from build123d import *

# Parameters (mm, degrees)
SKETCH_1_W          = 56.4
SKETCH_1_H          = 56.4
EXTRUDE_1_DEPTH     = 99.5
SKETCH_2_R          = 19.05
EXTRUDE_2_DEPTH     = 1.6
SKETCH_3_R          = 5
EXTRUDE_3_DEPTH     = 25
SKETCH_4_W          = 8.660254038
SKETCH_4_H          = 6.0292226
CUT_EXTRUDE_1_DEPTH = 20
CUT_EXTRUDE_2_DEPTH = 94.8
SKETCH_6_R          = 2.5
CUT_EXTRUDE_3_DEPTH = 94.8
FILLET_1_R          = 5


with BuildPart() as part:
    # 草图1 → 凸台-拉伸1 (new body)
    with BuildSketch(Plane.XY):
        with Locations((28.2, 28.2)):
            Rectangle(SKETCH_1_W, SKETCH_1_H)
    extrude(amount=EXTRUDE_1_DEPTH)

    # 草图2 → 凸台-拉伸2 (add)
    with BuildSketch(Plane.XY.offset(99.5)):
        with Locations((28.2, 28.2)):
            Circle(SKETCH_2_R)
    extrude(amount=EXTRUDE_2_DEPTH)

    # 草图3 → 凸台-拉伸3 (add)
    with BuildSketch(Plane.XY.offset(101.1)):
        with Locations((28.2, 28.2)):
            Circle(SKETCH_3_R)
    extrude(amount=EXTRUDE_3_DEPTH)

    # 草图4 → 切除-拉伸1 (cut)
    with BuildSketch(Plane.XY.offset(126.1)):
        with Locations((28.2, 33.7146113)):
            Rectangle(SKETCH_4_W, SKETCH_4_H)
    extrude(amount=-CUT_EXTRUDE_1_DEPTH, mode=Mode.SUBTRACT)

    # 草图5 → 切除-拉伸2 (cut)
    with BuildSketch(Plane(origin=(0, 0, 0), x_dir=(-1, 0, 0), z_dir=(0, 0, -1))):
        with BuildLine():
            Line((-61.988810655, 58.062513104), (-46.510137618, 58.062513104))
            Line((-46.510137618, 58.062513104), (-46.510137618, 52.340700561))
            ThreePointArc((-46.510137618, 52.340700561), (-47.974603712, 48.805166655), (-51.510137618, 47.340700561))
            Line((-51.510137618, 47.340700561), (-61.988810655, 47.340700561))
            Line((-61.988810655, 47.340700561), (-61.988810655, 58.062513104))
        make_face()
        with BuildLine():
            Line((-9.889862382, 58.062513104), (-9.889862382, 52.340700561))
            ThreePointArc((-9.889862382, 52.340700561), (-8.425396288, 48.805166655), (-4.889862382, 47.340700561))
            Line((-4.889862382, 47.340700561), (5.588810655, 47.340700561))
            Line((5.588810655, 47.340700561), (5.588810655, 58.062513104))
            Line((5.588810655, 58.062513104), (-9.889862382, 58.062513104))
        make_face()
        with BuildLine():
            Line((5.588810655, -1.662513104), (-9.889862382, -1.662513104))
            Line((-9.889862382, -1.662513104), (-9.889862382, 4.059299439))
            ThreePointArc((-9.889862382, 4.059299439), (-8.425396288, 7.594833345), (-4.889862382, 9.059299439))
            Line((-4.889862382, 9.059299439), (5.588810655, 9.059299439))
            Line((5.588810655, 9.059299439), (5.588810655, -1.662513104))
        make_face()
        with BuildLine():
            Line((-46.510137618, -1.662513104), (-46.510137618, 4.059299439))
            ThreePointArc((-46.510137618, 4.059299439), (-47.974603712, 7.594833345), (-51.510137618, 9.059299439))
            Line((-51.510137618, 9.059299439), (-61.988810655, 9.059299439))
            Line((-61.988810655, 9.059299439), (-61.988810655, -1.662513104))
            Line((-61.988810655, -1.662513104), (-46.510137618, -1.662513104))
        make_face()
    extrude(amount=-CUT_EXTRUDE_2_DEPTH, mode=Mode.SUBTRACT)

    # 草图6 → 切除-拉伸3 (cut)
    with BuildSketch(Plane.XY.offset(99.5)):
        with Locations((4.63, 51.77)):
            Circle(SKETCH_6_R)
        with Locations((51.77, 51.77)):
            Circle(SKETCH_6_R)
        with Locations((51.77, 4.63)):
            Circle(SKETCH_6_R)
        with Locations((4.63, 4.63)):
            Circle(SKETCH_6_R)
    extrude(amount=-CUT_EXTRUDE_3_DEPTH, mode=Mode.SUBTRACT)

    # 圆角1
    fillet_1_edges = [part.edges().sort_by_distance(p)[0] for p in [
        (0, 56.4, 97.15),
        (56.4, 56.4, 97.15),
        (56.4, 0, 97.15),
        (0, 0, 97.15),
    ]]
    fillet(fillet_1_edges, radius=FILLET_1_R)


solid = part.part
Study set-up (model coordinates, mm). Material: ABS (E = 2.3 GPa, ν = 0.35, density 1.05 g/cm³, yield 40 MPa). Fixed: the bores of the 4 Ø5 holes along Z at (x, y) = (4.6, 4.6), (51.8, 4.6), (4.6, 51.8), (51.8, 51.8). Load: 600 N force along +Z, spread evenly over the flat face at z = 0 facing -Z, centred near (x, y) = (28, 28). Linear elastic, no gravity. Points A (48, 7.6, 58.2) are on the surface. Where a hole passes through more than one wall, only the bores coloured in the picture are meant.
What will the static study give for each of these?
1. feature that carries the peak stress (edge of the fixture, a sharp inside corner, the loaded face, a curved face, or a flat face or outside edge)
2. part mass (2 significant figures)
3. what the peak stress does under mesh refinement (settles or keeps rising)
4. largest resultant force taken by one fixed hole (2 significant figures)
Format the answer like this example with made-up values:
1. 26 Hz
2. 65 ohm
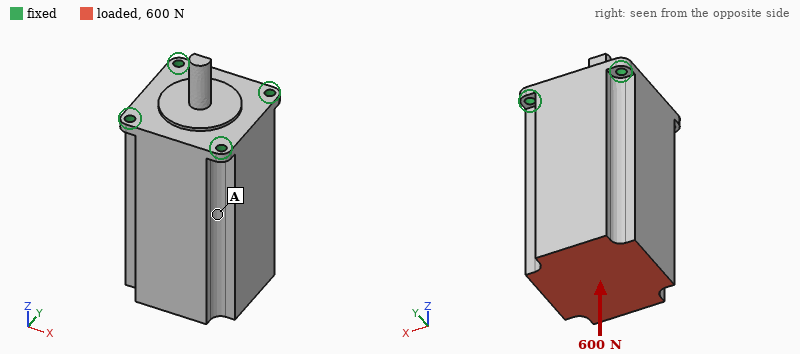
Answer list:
1. edge of the fixture
2. 300 g
3. keeps rising
4. 160 N
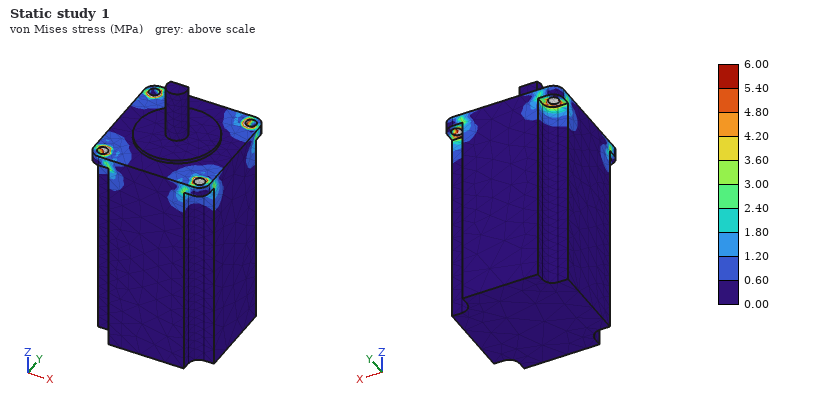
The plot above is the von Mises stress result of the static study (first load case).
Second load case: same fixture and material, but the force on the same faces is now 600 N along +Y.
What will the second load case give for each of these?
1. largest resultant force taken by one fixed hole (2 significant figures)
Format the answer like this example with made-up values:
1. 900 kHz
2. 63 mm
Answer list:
1. 700 N
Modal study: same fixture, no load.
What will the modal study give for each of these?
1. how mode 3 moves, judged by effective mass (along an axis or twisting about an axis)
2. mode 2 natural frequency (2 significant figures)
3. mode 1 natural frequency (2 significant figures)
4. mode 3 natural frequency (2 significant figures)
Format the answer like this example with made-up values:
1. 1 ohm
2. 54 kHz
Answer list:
1. along Z
2. 560 Hz
3. 550 Hz
4. 1500 Hz
